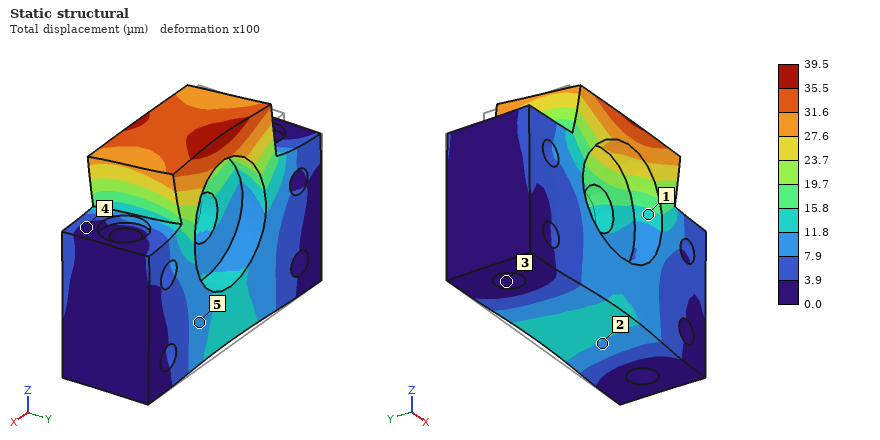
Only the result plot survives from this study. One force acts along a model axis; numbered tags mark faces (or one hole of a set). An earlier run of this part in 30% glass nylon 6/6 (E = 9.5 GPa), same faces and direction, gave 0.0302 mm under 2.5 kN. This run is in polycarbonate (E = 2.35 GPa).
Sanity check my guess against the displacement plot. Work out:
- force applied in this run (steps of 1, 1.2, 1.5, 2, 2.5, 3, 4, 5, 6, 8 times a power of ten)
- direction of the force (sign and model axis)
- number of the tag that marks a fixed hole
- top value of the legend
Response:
800 N
-Y
3
39.5 µm
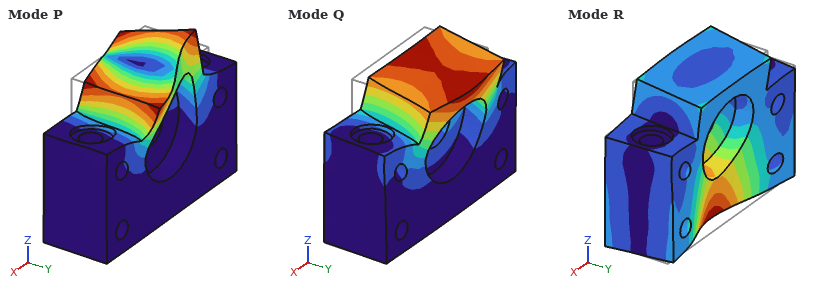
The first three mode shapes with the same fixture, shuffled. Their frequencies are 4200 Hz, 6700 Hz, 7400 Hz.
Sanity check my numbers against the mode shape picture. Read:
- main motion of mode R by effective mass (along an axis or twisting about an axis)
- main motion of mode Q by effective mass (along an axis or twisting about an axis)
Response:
along Y
along Y
